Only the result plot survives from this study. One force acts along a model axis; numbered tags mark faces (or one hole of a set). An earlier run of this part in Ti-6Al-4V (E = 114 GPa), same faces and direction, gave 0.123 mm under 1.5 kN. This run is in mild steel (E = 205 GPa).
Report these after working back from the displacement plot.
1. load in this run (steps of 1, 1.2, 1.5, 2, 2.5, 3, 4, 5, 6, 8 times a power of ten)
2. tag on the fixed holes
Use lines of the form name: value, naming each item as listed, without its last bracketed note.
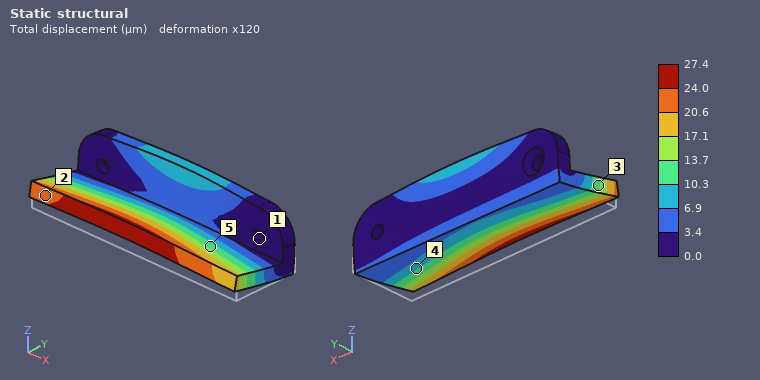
load in this run: 600 N
tag on the fixed holes: 1
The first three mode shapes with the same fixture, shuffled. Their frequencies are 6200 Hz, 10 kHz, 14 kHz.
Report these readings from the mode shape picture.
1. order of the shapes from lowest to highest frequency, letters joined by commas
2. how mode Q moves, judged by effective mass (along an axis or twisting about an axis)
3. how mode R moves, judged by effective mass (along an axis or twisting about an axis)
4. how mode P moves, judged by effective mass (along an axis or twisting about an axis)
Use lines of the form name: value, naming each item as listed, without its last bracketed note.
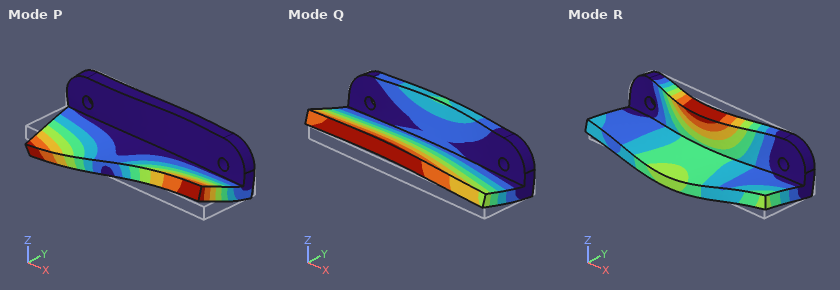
order of the shapes from lowest to highest frequency, letters joined by commas: Q, P, R
how mode Q moves, judged by effective mass: along Z
how mode R moves, judged by effective mass: along Y
how mode P moves, judged by effective mass: twisting about Y
